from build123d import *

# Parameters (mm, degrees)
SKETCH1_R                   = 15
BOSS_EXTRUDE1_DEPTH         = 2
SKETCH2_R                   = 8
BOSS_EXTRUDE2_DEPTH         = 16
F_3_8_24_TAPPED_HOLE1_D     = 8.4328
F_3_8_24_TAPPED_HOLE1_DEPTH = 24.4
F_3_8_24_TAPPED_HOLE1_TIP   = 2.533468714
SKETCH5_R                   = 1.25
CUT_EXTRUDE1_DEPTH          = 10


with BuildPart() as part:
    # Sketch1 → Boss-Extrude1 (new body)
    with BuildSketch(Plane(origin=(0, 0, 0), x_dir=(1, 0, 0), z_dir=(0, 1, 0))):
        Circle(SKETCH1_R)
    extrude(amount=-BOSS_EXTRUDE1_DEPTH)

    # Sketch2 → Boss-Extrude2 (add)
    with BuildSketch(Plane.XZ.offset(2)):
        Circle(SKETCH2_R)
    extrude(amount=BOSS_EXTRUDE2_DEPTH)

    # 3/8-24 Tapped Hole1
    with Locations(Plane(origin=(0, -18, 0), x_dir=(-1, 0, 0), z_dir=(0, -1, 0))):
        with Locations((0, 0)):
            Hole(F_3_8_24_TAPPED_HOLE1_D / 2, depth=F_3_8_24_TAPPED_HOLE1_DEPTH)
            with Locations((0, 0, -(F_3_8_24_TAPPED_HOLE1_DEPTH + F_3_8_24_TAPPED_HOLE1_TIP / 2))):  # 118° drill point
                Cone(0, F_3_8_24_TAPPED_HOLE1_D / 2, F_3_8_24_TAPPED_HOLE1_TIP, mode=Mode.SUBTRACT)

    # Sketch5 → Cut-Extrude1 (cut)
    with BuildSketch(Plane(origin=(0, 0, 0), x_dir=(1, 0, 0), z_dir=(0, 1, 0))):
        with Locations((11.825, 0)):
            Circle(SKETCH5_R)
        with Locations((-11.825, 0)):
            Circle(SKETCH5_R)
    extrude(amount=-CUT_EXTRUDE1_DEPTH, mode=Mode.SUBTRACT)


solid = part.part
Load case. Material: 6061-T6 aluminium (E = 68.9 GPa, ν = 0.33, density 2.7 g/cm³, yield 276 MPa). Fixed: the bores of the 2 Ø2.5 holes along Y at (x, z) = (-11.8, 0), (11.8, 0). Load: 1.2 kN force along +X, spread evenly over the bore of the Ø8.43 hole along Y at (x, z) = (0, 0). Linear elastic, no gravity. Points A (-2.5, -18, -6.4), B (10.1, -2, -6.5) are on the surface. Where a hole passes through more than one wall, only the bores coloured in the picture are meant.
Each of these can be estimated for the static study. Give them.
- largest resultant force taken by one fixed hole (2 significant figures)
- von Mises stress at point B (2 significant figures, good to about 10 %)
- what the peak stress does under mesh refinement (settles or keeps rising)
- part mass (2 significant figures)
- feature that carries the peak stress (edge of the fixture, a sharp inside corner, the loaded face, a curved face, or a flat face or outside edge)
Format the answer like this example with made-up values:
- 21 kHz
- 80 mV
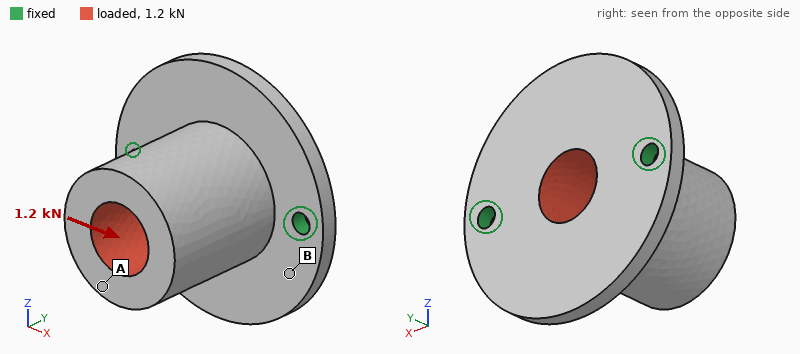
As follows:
- 780 N
- 25 MPa
- keeps rising
- 9.7 g
- edge of the fixture
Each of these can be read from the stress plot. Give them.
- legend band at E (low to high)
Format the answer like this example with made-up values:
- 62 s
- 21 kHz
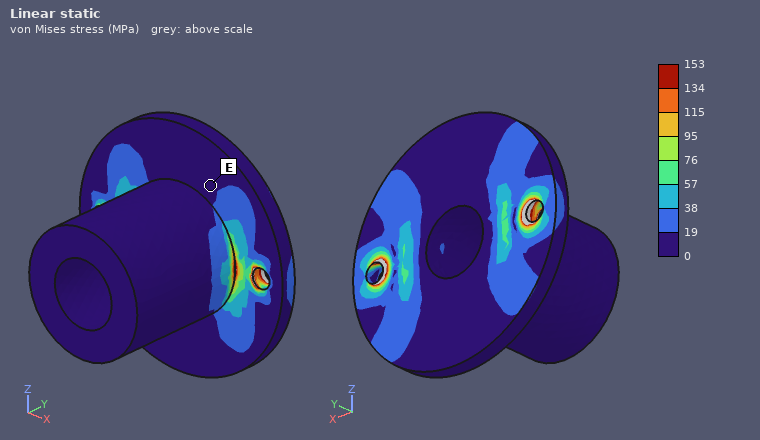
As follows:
- 0 to 19 MPa
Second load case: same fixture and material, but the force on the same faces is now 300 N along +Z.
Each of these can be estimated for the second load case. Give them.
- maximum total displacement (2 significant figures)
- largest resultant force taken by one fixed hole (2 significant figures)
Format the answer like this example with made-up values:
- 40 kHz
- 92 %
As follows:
- 95 µm
- 150 N
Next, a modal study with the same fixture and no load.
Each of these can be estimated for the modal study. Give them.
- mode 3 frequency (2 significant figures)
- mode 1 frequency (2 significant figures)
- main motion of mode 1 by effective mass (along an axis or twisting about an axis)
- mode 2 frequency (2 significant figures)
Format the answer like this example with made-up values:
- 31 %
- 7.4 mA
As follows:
- 12 kHz
- 3600 Hz
- along Z
- 12 kHz
